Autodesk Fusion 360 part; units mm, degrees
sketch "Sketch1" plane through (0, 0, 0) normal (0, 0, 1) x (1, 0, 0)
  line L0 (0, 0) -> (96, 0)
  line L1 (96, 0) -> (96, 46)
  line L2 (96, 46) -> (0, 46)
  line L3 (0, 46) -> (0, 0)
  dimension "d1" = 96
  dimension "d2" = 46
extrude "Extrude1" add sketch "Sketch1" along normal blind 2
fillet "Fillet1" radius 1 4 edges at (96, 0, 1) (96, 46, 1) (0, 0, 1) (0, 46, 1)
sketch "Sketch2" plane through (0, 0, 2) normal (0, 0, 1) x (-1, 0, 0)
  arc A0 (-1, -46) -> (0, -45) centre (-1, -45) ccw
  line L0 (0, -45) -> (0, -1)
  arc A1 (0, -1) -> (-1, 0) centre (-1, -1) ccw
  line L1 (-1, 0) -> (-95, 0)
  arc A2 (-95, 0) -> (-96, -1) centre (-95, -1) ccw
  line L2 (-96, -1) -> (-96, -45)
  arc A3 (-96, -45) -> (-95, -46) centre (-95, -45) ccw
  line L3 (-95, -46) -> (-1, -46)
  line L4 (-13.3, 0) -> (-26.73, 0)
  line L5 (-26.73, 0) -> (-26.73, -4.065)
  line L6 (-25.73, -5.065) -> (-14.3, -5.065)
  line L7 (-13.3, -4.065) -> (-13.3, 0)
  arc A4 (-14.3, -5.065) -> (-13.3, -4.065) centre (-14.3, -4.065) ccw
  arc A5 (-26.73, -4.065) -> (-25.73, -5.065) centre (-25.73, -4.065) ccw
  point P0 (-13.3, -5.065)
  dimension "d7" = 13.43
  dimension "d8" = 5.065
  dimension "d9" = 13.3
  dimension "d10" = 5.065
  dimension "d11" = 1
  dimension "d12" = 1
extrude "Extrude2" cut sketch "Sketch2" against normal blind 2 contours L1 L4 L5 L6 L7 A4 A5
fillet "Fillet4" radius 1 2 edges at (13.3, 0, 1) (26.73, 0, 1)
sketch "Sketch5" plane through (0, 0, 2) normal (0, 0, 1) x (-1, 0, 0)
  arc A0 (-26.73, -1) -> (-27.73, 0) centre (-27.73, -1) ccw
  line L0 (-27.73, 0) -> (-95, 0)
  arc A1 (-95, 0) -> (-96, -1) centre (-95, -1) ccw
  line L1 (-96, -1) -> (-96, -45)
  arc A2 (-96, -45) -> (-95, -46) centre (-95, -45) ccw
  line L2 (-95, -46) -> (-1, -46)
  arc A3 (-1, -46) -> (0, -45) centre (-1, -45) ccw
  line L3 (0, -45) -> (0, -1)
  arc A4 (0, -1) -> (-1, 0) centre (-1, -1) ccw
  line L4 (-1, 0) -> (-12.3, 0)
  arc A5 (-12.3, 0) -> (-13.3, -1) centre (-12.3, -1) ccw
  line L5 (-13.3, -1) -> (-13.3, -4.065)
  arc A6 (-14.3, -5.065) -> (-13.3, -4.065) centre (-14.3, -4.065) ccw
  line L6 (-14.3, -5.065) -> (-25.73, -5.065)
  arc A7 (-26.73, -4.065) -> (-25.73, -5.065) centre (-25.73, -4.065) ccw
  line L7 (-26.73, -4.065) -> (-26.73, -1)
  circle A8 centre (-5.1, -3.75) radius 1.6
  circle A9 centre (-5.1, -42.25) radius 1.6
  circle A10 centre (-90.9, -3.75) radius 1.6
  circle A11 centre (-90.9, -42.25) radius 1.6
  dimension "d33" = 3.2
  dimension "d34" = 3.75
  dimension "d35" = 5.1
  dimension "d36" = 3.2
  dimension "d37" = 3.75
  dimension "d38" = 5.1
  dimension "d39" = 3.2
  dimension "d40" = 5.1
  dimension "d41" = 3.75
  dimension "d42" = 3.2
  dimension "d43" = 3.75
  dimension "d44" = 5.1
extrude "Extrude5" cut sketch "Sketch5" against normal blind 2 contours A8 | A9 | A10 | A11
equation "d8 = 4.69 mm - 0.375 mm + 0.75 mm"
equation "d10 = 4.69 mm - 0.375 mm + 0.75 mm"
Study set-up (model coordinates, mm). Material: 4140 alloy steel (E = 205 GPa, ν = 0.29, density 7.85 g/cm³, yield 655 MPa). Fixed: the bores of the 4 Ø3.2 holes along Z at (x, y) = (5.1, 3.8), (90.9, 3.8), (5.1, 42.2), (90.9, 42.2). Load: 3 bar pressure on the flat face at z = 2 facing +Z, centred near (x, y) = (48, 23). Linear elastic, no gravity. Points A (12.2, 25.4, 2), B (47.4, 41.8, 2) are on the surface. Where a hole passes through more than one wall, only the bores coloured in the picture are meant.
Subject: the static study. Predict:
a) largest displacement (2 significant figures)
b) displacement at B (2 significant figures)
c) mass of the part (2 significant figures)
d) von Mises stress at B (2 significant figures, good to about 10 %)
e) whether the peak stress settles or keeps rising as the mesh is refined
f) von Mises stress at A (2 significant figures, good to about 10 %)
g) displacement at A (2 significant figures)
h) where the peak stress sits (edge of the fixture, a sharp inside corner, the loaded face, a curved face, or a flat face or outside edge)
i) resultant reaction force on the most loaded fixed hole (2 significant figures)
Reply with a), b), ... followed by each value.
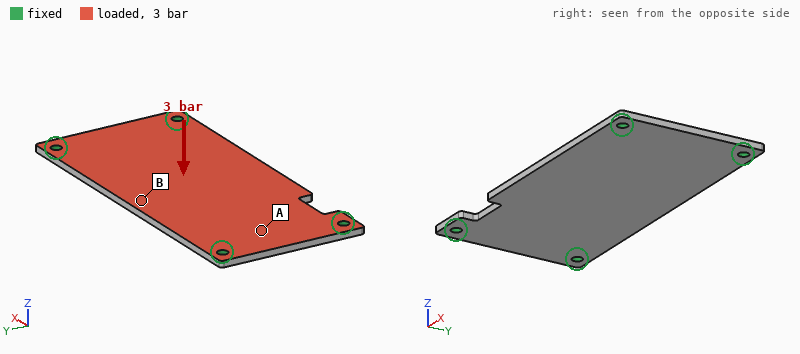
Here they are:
a) 0.40 mm
b) 0.38 mm
c) 68 g
d) 160 MPa
e) keeps rising
f) 90 MPa
g) 0.080 mm
h) edge of the fixture
i) 330 N
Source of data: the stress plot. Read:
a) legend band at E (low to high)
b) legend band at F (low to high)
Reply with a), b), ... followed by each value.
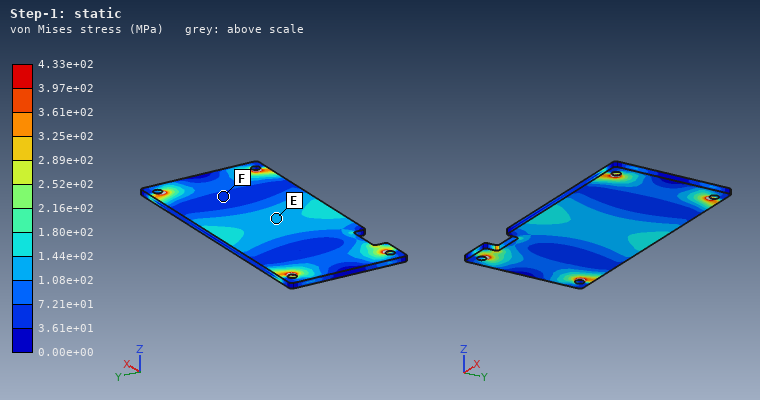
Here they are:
a) 1.08e+02 to 1.44e+02 MPa
b) 3.61e+01 to 7.21e+01 MPa
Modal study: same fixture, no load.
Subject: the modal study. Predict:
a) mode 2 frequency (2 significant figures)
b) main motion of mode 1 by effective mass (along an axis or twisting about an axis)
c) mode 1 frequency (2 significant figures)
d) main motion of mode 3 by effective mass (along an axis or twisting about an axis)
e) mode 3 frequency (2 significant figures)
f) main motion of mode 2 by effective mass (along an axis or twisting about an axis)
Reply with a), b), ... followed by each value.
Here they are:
a) 2200 Hz
b) along Z
c) 1300 Hz
d) twisting about Y
e) 3500 Hz
f) twisting about X
